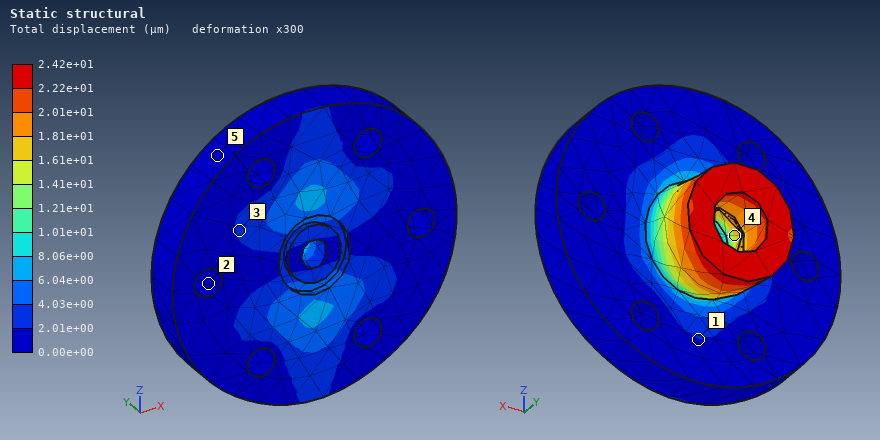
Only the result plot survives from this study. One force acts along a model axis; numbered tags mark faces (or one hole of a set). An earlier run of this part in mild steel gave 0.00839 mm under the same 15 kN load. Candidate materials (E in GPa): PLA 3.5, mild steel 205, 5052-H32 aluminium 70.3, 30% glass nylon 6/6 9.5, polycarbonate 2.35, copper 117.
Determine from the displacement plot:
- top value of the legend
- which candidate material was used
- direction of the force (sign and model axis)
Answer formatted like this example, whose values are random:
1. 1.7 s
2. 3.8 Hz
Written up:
1. 2.42e+01 µm
2. 5052-H32 aluminium
3. -Z
